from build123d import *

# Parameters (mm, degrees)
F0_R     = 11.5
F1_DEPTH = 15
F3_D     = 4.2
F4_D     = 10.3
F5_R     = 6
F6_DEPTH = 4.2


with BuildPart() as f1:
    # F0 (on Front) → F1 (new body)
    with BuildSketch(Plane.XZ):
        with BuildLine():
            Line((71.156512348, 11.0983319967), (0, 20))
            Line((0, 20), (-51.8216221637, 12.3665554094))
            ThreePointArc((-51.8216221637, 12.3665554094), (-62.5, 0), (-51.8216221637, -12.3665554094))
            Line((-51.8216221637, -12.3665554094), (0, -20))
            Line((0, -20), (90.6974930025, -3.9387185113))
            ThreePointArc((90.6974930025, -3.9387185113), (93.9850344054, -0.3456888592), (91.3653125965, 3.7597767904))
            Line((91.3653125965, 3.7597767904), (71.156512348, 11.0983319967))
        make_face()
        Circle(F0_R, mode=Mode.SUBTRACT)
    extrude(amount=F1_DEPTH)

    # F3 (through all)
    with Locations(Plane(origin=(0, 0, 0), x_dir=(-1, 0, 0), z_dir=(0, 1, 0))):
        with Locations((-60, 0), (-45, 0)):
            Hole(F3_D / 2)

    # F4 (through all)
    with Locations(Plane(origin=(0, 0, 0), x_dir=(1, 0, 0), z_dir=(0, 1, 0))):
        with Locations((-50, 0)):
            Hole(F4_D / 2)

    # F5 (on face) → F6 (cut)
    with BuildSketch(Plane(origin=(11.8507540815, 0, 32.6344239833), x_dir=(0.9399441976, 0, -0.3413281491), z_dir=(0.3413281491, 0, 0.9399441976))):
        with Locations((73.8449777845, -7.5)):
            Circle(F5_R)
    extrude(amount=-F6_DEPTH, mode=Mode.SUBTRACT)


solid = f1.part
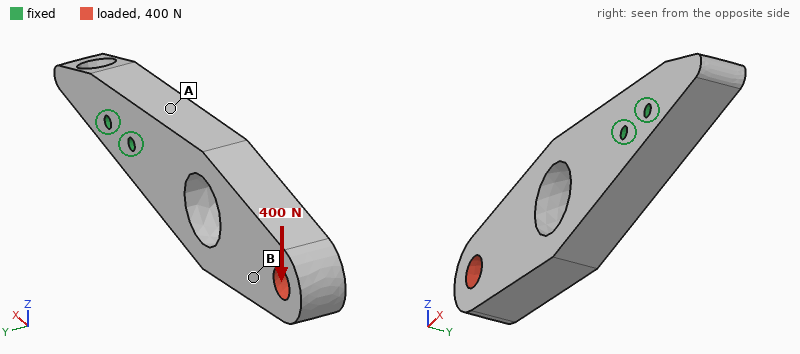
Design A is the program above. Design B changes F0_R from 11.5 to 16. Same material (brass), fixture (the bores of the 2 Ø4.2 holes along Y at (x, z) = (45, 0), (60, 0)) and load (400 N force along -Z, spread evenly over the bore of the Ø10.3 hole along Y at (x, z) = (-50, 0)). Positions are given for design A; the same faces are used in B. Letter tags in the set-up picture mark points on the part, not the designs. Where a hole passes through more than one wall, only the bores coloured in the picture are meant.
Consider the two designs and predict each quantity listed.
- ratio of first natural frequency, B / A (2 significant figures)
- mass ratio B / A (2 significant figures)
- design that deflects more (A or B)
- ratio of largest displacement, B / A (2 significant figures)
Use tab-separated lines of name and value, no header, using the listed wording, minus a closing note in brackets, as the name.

ratio of first natural frequency, B / A	0.84
mass ratio B / A	0.89
design that deflects more	B
ratio of largest displacement, B / A	1.5
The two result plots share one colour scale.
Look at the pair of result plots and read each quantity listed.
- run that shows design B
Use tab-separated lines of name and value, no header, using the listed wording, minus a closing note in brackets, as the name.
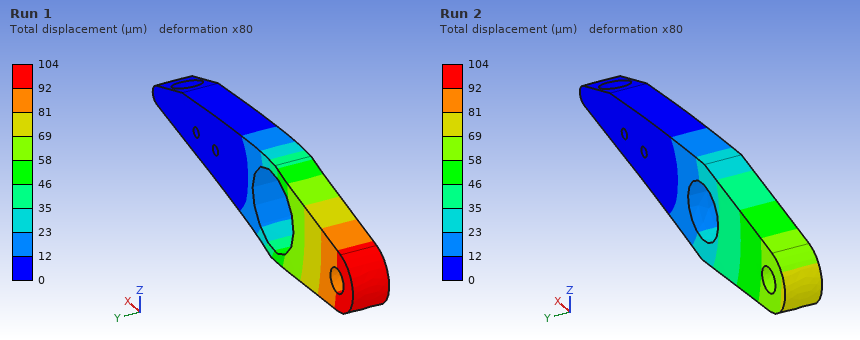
run that shows design B	Run 1
